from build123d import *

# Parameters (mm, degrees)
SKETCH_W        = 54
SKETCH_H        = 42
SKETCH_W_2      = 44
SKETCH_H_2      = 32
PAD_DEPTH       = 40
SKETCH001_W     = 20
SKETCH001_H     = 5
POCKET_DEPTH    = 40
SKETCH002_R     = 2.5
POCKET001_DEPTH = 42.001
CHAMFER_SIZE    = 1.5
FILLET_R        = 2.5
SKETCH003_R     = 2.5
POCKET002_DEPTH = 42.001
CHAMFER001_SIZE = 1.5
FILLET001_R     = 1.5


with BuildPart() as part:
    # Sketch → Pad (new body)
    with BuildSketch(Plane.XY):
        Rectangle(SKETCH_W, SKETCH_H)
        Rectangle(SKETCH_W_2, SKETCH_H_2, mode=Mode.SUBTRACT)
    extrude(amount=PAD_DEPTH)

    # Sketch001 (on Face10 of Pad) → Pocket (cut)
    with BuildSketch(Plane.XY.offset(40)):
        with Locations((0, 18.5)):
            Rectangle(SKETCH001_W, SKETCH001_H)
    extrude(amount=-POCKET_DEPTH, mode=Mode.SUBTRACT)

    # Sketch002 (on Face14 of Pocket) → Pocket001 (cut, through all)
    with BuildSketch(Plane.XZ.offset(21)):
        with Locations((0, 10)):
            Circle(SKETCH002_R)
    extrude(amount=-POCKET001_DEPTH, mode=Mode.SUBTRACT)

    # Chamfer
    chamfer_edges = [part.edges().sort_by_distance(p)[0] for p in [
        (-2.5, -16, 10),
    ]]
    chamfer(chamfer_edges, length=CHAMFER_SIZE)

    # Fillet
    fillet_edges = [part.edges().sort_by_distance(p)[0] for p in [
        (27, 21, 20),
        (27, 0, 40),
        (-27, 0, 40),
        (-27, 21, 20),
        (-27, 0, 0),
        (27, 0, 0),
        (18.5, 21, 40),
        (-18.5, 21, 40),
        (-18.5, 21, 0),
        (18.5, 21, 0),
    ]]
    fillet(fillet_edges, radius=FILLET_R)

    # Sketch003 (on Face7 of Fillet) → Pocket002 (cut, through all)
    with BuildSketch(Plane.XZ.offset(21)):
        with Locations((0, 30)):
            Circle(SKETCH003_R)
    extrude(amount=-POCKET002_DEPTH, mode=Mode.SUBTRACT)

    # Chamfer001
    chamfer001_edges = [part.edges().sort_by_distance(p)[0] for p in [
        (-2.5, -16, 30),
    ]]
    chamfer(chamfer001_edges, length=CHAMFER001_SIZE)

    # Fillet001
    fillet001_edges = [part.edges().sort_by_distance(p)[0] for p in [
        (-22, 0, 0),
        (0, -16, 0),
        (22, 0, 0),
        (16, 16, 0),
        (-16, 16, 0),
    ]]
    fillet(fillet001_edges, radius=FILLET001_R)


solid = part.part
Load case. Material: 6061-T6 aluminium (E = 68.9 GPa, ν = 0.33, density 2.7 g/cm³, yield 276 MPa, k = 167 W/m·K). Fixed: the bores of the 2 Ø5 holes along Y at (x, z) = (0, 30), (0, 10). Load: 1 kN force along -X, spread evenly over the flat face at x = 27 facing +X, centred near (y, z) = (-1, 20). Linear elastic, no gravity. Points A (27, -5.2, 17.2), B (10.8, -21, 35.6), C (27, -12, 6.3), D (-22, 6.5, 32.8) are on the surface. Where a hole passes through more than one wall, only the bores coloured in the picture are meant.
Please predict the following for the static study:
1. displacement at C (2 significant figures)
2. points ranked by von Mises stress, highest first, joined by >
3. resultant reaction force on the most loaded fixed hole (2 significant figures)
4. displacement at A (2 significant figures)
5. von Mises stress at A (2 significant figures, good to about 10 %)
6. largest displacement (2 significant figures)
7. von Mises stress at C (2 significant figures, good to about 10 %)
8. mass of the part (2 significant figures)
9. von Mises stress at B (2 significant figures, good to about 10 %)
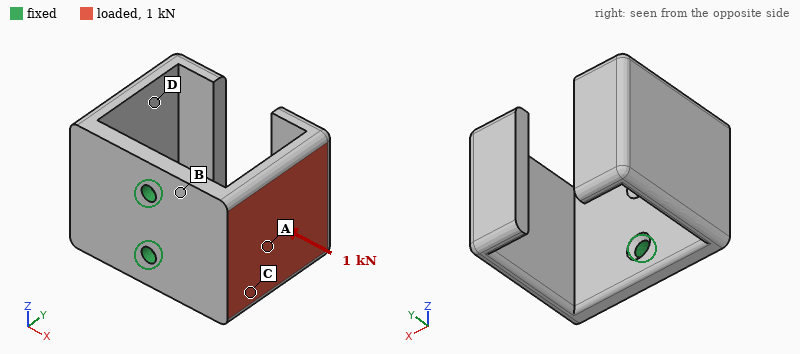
0.26 mm
B > C > A > D
510 N
0.33 mm
38 MPa
0.79 mm
68 MPa
80 g
96 MPa
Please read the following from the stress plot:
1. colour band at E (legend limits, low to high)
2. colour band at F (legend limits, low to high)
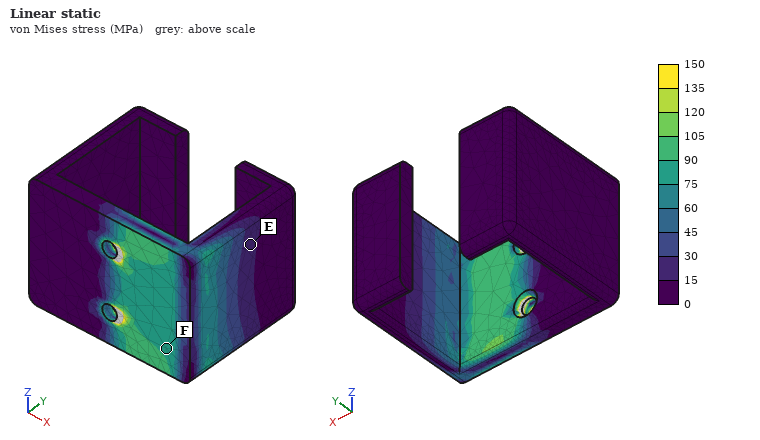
15 to 30 MPa
75 to 90 MPa
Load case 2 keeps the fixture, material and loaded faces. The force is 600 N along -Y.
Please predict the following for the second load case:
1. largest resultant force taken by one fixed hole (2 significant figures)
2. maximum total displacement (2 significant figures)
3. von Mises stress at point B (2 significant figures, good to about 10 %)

300 N
0.36 mm
56 MPa
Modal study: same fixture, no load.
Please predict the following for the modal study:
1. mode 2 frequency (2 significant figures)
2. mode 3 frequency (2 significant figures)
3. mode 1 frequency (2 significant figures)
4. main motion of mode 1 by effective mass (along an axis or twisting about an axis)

1000 Hz
1700 Hz
970 Hz
along X
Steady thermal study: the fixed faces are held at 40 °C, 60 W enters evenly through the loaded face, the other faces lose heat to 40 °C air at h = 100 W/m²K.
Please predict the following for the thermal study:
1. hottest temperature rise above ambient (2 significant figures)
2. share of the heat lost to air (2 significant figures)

50 K
32 %
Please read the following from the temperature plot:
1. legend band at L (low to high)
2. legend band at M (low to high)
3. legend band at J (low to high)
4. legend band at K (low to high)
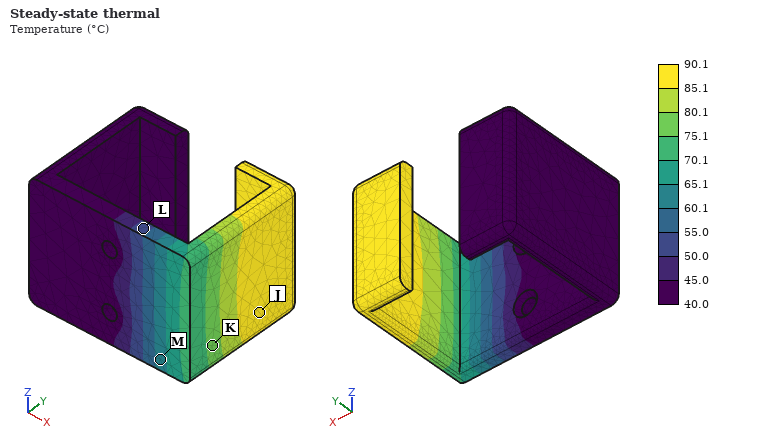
50.0 to 55.0 °C
60.1 to 65.1 °C
85.1 to 90.1 °C
75.1 to 80.1 °C
